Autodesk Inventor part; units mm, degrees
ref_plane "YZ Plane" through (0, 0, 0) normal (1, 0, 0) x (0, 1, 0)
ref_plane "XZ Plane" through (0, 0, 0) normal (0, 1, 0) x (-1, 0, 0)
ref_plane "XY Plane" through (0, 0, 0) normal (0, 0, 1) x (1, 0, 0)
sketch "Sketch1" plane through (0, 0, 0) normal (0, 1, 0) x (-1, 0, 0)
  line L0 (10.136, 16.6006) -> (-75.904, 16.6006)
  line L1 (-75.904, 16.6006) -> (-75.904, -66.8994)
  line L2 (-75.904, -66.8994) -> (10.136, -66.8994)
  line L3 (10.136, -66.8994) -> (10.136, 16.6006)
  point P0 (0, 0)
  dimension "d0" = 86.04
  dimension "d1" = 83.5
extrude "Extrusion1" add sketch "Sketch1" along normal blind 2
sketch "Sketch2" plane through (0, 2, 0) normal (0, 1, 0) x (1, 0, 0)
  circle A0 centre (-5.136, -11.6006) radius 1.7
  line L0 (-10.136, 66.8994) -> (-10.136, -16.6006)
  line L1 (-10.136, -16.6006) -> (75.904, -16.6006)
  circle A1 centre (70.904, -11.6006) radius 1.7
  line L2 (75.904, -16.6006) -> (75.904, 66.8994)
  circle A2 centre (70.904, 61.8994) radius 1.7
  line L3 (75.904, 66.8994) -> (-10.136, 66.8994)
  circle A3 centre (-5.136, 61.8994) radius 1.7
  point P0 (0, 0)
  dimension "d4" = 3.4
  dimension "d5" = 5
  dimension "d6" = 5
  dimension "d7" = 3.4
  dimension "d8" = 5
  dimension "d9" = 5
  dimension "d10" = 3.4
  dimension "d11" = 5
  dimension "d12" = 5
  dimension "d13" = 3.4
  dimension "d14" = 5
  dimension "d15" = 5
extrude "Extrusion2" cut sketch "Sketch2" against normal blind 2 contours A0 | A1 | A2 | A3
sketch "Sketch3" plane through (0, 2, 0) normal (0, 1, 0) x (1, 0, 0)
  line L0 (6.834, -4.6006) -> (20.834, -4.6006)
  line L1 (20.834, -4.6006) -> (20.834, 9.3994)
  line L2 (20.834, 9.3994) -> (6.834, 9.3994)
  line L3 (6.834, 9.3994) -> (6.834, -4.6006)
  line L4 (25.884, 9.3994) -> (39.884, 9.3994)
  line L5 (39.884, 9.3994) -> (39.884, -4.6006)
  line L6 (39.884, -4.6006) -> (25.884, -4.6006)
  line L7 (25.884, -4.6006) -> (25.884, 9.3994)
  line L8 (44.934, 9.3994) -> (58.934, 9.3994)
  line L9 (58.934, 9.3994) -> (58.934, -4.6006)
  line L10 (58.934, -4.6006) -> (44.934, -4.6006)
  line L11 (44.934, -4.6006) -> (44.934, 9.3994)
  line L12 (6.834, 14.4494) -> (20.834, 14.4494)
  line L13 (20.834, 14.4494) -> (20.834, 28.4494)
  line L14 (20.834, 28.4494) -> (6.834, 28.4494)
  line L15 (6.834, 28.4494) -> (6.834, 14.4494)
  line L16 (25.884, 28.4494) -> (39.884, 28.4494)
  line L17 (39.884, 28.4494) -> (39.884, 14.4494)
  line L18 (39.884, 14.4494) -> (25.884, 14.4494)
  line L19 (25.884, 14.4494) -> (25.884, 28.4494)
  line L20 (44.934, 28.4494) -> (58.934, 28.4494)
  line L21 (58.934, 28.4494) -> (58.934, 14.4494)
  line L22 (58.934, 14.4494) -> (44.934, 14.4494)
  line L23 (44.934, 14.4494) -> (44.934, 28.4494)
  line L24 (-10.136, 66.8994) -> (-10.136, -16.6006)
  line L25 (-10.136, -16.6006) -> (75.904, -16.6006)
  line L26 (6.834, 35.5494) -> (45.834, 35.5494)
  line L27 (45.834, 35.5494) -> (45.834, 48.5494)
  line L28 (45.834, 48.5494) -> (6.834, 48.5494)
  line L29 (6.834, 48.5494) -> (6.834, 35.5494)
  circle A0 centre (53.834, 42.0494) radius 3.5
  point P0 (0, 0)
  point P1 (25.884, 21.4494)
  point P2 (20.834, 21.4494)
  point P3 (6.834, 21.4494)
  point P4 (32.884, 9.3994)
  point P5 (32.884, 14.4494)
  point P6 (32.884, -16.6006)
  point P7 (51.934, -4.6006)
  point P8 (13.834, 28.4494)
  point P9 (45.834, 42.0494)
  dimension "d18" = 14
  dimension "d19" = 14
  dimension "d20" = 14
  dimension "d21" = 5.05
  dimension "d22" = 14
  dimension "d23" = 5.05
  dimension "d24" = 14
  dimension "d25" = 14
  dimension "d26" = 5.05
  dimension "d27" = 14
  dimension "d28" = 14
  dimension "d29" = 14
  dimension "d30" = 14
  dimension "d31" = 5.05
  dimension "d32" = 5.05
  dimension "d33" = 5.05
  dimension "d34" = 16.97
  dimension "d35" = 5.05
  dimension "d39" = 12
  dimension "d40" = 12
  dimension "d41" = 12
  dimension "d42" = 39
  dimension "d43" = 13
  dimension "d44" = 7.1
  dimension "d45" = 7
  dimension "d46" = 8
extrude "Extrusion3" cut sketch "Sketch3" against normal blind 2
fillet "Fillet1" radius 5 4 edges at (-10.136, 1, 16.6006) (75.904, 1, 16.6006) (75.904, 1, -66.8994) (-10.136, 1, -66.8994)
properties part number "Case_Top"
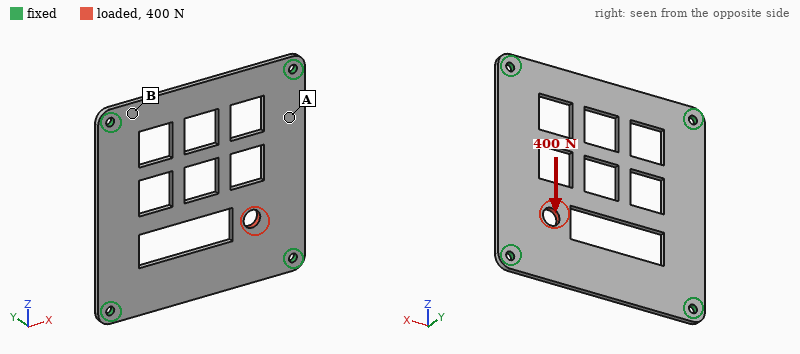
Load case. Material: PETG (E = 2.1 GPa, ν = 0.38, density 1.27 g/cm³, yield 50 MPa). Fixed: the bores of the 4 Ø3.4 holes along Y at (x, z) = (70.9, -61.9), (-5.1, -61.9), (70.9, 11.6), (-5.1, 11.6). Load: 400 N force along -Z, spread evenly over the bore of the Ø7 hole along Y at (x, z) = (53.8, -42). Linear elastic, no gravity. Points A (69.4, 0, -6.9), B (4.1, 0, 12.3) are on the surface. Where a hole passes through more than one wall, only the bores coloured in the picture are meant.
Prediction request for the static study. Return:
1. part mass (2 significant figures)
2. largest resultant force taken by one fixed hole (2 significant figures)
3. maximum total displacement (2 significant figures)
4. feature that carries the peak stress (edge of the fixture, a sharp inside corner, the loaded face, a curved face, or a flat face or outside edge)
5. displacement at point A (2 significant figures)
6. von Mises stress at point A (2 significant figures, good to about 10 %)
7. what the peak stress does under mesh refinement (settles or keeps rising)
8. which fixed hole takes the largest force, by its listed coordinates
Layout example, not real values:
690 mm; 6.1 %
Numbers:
14 g; 240 N; 0.21 mm; edge of the fixture; 0.057 mm; 4.1 MPa; keeps rising; (70.9, -61.9)
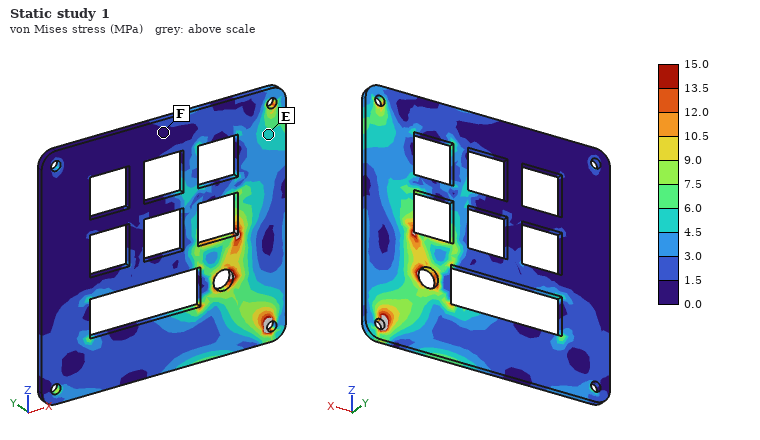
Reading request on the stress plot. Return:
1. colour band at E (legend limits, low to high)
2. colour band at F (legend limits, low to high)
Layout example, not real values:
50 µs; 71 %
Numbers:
4.5 to 6.0 MPa; 0.0 to 1.5 MPa
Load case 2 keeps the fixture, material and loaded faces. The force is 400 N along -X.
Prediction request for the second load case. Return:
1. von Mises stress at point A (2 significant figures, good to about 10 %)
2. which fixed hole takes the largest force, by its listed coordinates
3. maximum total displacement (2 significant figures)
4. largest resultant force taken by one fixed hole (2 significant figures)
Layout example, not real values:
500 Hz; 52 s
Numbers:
2.5 MPa; (70.9, -61.9); 0.26 mm; 220 N
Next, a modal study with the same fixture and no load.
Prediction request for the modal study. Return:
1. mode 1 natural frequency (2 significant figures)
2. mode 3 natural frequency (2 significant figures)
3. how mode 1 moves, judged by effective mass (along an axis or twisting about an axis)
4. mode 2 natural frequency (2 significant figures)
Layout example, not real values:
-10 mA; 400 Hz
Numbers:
320 Hz; 520 Hz; along Y; 500 Hz
